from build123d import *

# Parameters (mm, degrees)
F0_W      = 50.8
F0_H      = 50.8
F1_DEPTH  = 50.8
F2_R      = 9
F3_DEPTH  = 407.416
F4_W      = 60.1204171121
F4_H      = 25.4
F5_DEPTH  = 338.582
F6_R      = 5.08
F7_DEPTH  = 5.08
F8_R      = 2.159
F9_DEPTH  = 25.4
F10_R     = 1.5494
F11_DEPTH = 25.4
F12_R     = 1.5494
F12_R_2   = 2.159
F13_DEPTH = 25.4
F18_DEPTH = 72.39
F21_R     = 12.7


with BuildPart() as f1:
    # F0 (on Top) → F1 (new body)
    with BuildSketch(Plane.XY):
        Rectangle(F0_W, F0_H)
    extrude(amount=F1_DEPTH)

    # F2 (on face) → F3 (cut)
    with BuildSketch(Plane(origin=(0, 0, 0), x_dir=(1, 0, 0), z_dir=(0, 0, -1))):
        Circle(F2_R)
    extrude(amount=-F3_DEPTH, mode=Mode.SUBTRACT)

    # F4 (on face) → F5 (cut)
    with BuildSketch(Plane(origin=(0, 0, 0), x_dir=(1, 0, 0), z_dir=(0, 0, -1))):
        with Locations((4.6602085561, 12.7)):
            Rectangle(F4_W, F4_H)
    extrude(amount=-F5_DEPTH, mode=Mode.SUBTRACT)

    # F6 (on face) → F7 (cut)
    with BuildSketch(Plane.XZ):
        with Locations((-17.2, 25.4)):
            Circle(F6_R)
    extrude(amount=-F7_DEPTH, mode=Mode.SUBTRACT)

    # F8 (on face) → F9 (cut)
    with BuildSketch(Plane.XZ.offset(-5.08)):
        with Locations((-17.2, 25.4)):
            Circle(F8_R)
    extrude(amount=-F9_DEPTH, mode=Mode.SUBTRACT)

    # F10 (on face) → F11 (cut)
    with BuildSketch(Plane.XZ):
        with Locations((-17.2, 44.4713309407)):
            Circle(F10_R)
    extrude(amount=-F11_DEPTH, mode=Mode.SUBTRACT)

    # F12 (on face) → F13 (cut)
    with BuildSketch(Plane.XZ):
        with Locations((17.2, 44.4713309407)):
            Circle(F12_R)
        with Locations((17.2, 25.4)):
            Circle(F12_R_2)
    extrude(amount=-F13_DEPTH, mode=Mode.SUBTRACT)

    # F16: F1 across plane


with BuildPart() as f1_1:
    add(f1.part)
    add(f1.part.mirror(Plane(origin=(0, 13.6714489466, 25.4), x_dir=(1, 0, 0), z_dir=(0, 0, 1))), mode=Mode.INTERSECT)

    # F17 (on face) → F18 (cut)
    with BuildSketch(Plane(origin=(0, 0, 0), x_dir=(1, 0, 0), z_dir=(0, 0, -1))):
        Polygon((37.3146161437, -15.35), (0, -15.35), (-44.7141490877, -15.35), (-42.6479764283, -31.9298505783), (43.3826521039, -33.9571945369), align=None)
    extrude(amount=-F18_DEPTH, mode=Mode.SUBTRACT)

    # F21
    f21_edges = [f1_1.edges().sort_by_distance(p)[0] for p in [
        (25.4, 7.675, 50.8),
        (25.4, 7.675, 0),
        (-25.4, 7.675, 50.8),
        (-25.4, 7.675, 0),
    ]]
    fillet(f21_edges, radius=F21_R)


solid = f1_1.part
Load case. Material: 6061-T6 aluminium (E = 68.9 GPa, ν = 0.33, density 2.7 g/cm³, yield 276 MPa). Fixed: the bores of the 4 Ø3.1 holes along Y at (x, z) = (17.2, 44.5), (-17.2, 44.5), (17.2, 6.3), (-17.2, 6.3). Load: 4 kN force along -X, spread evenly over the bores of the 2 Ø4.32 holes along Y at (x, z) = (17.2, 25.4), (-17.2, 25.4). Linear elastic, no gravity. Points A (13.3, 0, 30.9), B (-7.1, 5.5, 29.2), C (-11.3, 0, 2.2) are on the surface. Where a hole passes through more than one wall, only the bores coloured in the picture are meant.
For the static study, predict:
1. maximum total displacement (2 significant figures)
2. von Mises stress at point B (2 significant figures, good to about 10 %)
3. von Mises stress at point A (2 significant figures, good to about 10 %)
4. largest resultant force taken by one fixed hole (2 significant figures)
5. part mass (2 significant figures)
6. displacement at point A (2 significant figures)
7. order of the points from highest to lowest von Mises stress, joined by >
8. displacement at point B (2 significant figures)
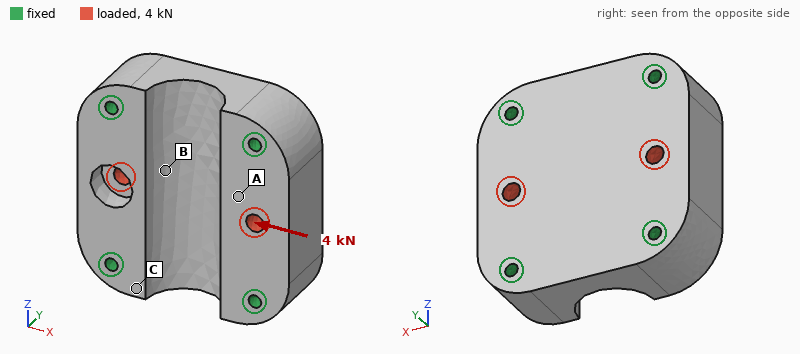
5.5 µm
5.6 MPa
9.2 MPa
1.1 kN
80 g
4.0 µm
A > B > C
2.5 µm
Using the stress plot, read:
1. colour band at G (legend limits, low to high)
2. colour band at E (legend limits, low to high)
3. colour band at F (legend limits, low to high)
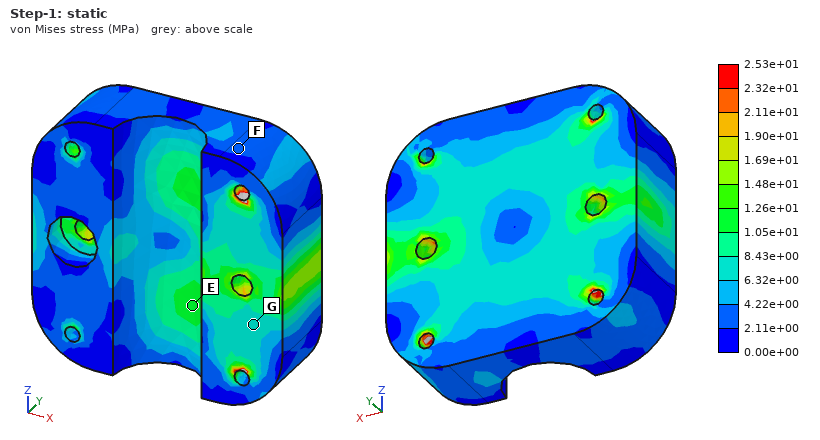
6.32e+00 to 8.43e+00 MPa
1.05e+01 to 1.26e+01 MPa
2.11e+00 to 4.22e+00 MPa
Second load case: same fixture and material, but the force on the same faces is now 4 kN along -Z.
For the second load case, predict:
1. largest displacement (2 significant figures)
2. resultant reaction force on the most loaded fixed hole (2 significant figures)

2.0 µm
1.2 kN
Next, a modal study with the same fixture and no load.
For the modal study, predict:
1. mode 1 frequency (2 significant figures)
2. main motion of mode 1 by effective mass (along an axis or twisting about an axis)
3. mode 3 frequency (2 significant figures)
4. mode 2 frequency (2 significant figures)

24 kHz
along Y
31 kHz
29 kHz
